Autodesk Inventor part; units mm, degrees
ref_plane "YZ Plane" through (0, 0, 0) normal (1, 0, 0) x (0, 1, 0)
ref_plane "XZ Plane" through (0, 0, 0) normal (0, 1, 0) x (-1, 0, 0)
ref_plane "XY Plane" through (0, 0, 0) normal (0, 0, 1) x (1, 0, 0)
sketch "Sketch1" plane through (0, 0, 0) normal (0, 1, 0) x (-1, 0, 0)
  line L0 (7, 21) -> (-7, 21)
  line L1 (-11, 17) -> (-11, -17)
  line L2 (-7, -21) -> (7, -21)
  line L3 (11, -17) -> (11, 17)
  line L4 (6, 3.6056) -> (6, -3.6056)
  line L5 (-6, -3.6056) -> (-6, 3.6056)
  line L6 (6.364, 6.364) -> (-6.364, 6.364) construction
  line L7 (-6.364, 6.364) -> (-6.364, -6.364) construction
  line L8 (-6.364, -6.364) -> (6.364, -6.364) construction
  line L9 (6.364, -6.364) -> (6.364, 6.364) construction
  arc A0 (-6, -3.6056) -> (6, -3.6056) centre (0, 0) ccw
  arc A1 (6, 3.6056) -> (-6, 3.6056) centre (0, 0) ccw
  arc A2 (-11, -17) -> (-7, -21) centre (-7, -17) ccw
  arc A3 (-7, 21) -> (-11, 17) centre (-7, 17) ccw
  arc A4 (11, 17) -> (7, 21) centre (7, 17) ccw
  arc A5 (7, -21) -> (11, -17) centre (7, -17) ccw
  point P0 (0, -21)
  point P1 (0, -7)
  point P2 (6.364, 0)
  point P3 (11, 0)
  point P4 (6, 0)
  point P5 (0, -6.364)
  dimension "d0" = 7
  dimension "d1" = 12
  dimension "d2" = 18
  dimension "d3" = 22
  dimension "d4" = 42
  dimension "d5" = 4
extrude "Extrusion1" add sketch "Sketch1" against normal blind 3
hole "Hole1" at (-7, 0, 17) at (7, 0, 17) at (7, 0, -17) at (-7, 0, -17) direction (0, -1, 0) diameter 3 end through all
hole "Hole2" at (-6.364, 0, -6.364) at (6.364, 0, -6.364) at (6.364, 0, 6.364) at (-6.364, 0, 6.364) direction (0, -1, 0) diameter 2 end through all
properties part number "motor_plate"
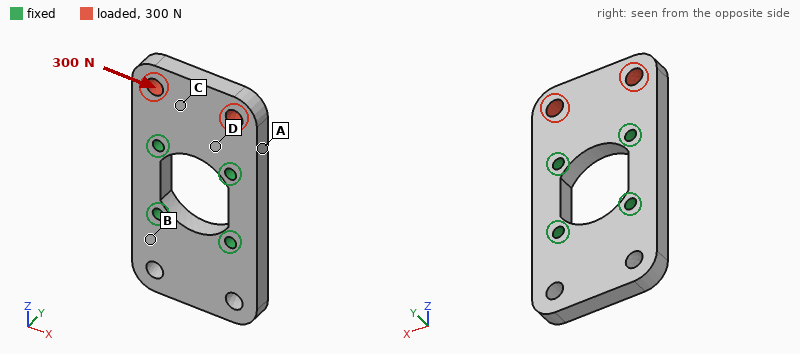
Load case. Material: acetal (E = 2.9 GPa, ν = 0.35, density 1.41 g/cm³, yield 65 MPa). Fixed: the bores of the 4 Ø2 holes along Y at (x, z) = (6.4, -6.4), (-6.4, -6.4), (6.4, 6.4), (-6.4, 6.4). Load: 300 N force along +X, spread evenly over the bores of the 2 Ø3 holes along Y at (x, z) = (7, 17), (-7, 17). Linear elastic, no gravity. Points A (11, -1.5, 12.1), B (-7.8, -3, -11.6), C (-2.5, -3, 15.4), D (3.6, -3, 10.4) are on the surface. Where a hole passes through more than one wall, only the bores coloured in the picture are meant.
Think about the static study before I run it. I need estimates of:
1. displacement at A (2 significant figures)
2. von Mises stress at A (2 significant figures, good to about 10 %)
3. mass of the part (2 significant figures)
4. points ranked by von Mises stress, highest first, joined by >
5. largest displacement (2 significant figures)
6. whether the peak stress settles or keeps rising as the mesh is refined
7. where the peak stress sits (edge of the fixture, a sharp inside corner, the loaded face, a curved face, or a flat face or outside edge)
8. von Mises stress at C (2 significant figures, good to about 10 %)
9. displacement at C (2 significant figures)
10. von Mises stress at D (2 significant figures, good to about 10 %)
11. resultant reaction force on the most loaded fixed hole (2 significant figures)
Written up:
0.061 mm
5.5 MPa
3.1 g
D > C > A > B
0.11 mm
keeps rising
edge of the fixture
9.3 MPa
0.066 mm
12 MPa
230 N
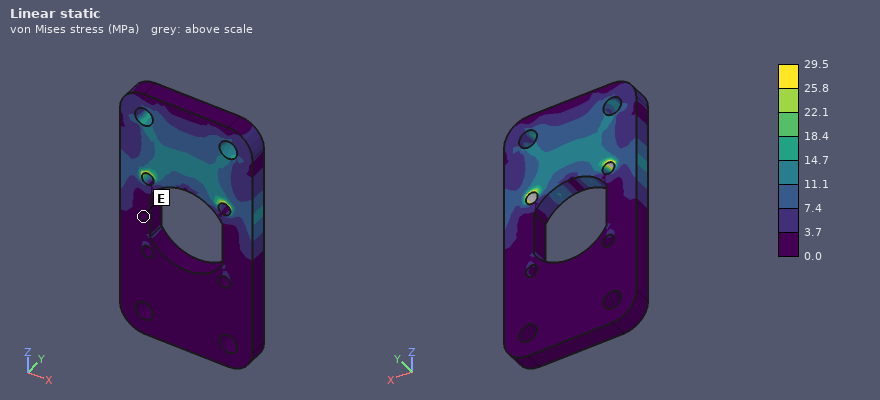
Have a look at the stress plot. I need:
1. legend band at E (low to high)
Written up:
0.0 to 3.7 MPa
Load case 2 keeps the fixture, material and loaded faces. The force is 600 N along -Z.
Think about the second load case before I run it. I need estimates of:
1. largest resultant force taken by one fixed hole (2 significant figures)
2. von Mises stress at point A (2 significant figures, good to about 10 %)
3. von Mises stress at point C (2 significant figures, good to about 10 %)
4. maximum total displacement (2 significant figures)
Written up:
280 N
11 MPa
5.6 MPa
68 µm
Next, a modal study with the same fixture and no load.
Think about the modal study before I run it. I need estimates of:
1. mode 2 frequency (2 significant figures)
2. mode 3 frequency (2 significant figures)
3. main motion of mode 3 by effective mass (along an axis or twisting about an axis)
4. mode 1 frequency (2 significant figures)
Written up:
3000 Hz
5900 Hz
twisting about Z
3000 Hz
